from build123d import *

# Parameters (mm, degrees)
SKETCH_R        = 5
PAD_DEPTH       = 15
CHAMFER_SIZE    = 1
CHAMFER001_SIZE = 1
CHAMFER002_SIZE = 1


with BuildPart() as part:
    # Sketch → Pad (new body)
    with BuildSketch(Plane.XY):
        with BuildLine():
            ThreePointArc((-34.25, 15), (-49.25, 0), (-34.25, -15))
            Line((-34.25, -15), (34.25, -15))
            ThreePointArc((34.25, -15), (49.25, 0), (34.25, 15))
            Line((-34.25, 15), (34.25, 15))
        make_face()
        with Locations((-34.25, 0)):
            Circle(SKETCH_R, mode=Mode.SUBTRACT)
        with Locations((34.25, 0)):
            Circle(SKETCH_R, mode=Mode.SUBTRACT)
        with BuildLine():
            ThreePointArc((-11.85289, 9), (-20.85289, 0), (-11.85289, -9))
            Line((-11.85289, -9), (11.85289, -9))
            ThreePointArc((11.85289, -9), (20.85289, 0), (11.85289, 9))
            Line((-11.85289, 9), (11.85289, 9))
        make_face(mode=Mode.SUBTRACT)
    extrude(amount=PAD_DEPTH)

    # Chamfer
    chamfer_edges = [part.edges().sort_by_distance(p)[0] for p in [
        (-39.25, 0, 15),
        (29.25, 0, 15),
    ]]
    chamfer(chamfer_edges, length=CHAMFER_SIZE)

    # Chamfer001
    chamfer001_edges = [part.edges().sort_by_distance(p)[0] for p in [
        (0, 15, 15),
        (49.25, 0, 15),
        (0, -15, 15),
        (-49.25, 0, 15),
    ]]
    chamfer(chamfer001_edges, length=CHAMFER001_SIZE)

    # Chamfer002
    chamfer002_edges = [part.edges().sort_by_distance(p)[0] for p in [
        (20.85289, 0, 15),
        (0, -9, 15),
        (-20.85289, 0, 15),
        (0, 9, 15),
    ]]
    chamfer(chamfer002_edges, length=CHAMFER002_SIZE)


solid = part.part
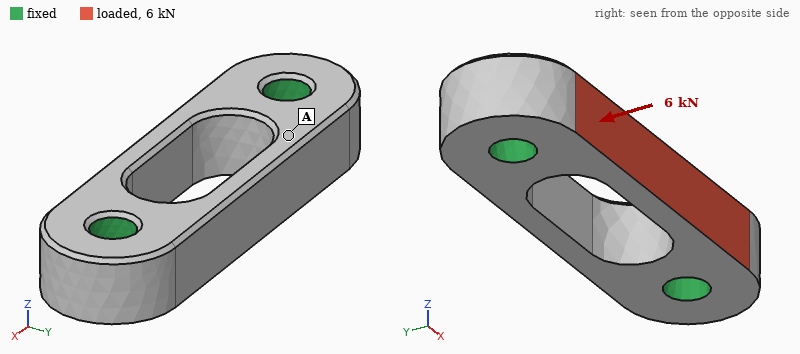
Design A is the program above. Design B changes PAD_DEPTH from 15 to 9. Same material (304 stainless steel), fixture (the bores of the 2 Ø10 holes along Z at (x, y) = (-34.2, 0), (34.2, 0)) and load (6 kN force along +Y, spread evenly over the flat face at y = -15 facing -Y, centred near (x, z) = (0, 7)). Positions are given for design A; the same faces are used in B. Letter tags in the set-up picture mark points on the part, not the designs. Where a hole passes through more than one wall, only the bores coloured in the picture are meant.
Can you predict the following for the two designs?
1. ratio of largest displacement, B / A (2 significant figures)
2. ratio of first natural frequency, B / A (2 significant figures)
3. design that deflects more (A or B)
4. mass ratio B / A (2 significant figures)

1.7
0.74
B
0.60
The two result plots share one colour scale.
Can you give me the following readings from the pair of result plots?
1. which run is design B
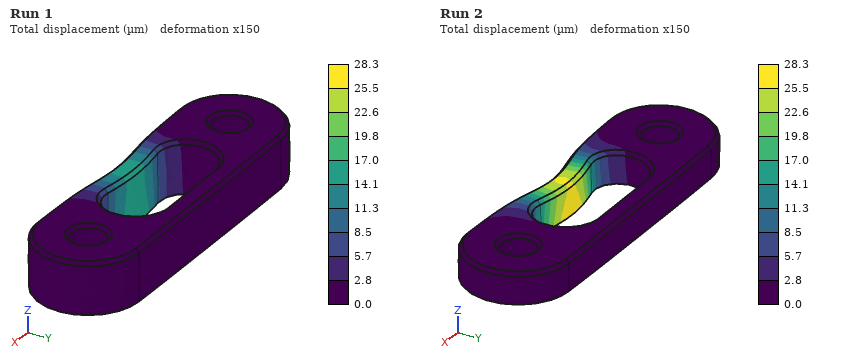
Run 2
